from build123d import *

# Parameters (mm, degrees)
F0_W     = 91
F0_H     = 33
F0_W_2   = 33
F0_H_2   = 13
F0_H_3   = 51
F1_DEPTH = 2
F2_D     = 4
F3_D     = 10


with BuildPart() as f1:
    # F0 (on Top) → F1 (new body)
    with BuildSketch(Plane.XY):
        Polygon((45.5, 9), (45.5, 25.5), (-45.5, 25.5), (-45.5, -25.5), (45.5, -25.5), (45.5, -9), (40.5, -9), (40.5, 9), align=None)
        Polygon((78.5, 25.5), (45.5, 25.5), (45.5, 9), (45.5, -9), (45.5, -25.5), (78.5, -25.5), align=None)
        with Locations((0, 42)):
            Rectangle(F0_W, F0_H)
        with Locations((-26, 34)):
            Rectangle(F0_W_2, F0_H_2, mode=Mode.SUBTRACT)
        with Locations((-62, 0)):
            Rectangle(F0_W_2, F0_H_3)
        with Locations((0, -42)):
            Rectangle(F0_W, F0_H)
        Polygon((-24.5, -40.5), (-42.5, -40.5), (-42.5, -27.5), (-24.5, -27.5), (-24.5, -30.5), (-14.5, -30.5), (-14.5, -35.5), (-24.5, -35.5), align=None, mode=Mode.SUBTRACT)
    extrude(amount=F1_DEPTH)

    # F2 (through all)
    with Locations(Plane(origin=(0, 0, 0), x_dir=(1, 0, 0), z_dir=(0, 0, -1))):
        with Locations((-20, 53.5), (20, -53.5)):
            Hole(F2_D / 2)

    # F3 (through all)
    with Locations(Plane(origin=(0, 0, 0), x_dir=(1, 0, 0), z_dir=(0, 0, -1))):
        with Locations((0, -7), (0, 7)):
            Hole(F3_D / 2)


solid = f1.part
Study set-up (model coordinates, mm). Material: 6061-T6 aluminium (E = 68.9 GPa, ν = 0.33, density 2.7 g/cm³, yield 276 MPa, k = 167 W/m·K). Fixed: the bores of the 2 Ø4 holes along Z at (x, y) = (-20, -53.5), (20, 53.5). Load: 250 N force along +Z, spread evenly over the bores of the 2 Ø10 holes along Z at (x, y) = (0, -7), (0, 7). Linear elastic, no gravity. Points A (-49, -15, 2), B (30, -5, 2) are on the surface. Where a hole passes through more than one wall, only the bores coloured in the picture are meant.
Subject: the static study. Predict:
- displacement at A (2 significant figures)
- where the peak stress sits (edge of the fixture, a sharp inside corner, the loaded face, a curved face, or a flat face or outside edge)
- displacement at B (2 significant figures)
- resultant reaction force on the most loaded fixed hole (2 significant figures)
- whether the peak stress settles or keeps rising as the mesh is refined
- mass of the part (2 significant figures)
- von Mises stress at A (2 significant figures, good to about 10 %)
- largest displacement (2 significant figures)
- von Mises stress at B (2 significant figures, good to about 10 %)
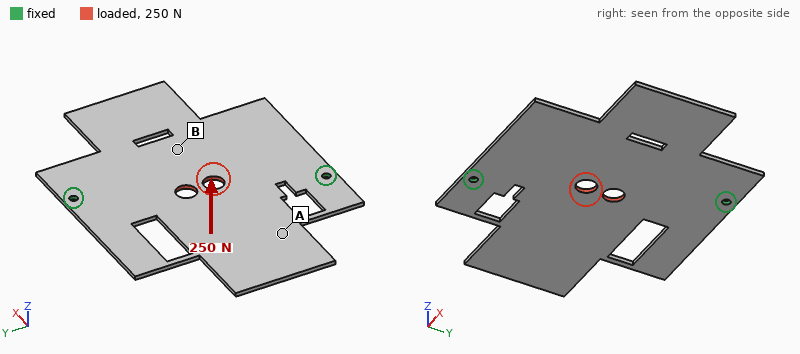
0.49 mm
edge of the fixture
0.66 mm
130 N
keeps rising
70 g
17 MPa
0.91 mm
44 MPa
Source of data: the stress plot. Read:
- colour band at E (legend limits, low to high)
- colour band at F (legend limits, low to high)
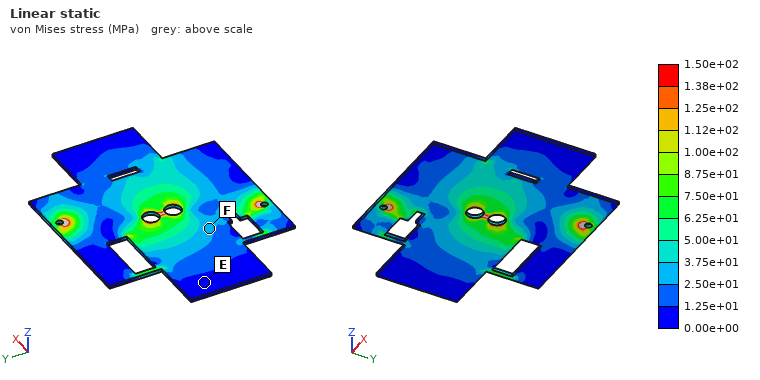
0.00e+00 to 1.25e+01 MPa
2.50e+01 to 3.75e+01 MPa
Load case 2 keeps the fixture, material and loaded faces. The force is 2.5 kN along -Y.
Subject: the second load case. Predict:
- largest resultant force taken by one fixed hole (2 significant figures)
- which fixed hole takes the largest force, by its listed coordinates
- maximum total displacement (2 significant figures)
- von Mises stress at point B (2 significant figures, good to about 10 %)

1.6 kN
(20, 53.5)
35 µm
8.2 MPa
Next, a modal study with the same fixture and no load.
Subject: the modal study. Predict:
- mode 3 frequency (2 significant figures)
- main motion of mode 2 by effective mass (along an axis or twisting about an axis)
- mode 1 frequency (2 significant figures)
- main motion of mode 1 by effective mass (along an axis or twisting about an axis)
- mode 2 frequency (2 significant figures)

670 Hz
along Z
210 Hz
twisting about Y
310 Hz
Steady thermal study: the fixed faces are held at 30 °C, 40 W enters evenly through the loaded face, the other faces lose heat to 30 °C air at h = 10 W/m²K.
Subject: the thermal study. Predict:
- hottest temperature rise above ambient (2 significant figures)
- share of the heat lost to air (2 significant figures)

82 K
27 %
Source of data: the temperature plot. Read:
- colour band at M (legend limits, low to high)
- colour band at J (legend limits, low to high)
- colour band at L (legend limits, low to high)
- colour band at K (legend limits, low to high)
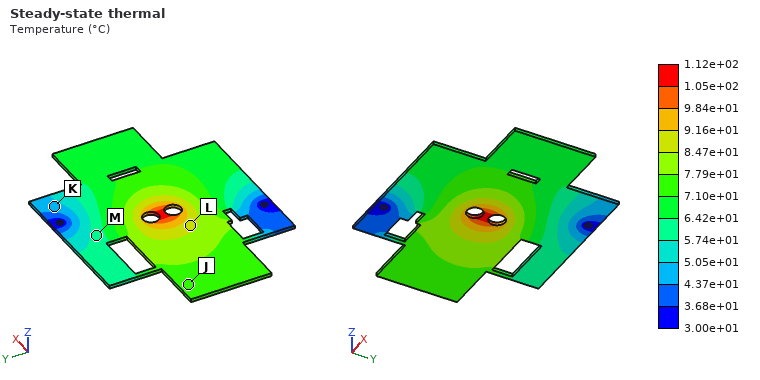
5.74e+01 to 6.42e+01 °C
7.10e+01 to 7.79e+01 °C
8.47e+01 to 9.16e+01 °C
4.37e+01 to 5.05e+01 °C
